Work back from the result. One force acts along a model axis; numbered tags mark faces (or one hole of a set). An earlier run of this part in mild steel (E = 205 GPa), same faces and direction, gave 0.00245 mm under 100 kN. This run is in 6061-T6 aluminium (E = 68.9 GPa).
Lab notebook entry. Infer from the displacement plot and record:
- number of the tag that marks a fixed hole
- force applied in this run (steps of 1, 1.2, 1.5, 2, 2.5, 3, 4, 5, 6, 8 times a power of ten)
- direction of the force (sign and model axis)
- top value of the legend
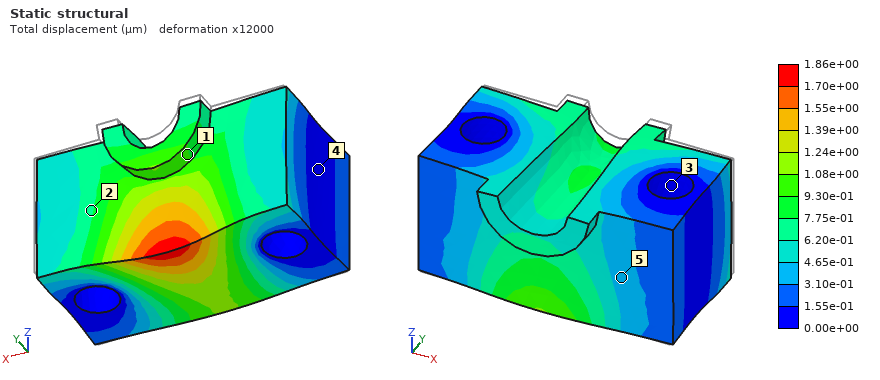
3
25 kN
-Y
1.86e+00 µm
